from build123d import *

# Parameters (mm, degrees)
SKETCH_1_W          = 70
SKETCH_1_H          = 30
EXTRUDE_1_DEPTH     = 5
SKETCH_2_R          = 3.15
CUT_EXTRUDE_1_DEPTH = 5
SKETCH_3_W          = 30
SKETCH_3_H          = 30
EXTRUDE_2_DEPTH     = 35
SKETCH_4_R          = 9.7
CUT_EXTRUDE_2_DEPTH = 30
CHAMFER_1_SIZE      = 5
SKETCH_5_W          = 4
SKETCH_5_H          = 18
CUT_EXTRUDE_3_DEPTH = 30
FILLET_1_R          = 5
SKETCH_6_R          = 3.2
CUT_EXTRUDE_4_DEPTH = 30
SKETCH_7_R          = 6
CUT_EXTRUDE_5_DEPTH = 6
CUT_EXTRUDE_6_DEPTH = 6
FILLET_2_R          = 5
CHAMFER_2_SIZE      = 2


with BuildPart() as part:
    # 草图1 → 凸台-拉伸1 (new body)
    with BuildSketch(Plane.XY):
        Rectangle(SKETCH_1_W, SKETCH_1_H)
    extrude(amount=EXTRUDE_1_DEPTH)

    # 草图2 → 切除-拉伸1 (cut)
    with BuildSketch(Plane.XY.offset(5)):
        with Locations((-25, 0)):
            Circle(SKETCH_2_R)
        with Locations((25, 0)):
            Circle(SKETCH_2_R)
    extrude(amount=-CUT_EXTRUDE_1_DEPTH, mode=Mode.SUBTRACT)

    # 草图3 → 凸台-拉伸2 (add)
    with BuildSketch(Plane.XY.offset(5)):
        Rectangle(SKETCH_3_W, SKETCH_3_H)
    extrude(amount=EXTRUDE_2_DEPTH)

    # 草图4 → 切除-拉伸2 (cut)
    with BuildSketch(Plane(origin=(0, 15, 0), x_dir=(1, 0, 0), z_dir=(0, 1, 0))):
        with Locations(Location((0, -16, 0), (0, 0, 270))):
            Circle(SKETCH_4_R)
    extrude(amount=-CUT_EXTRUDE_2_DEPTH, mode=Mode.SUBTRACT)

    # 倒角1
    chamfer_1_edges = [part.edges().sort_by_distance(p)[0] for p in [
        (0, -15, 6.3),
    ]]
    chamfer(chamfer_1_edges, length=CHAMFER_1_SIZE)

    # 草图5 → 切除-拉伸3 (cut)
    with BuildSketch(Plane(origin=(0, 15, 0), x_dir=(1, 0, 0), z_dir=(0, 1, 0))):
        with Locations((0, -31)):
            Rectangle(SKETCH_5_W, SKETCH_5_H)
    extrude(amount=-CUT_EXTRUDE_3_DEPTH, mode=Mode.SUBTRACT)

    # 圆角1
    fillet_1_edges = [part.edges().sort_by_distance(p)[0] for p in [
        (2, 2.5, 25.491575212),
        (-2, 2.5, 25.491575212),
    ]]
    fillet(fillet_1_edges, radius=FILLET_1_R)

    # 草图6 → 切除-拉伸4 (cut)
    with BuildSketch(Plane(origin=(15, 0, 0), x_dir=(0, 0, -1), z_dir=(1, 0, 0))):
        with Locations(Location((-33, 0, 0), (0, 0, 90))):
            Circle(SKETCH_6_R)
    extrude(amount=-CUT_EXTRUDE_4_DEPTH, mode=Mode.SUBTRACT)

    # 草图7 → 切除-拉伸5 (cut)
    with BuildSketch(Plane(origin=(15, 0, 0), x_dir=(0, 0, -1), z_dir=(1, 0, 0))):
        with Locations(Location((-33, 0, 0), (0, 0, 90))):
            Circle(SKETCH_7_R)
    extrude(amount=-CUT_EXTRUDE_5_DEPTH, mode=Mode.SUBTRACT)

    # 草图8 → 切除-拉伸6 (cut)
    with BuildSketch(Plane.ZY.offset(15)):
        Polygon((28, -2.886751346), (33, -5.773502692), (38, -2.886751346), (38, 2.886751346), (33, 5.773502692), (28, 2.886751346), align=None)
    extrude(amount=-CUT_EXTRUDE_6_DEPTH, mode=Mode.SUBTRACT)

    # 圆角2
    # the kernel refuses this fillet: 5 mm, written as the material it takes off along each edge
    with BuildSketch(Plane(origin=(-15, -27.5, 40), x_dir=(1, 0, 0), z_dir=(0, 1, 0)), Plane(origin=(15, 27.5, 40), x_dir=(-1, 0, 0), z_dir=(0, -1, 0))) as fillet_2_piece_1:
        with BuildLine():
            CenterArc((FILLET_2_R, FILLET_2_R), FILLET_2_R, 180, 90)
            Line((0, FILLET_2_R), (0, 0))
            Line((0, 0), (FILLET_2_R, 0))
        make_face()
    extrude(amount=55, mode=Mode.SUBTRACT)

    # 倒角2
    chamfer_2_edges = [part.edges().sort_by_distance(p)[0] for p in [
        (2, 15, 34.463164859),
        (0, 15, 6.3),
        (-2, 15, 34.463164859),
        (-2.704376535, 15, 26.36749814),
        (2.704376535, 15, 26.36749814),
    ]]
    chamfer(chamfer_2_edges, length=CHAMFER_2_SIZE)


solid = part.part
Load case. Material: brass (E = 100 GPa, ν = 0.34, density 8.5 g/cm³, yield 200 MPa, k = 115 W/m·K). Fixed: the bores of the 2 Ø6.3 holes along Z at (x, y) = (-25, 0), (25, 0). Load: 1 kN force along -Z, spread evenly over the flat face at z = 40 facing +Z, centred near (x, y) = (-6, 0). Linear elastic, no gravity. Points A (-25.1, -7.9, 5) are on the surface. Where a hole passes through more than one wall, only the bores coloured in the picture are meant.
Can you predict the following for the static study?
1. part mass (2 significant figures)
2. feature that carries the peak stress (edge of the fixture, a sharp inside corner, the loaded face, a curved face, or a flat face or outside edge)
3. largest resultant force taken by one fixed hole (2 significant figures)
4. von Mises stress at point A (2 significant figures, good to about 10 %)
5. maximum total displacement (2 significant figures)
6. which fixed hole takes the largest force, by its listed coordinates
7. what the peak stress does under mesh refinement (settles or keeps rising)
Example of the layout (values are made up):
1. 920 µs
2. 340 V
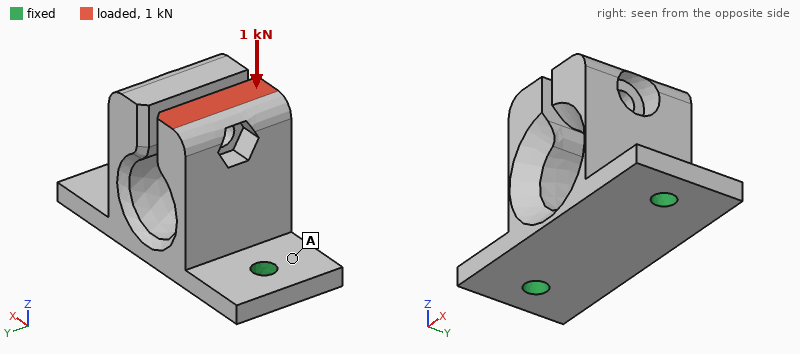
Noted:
1. 240 g
2. edge of the fixture
3. 730 N
4. 11 MPa
5. 78 µm
6. (-25, 0)
7. keeps rising
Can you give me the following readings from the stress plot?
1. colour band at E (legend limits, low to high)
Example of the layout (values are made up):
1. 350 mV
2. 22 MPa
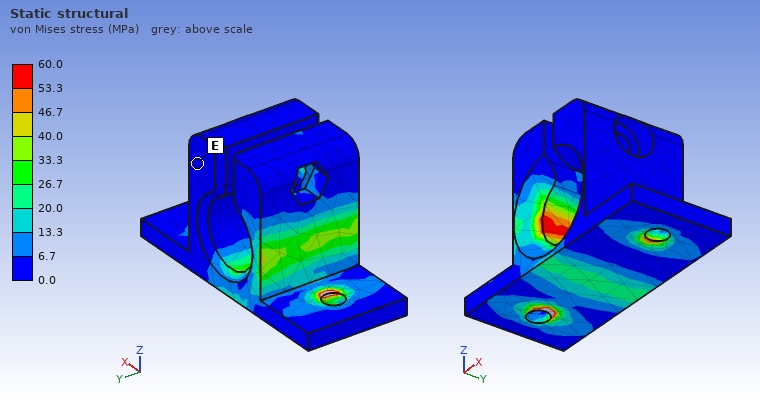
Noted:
1. 0.0 to 6.7 MPa
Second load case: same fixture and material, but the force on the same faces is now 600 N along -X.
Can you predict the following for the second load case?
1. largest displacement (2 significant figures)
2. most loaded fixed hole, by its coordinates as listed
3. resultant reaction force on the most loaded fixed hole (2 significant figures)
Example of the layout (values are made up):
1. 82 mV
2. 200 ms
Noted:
1. 0.18 mm
2. (25, 0)
3. 850 N
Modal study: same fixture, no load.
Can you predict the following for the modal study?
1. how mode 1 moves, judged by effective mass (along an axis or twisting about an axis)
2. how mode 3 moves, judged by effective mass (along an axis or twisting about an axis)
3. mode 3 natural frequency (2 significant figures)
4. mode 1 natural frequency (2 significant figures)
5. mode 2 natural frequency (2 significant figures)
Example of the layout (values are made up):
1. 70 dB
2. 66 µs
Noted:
1. along Y
2. along X
3. 2100 Hz
4. 1600 Hz
5. 1700 Hz
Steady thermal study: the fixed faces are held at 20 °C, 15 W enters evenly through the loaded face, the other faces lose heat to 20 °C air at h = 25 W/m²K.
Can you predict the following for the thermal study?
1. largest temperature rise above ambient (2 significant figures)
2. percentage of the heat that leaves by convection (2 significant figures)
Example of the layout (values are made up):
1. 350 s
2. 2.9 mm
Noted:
1. 29 K
2. 14 %
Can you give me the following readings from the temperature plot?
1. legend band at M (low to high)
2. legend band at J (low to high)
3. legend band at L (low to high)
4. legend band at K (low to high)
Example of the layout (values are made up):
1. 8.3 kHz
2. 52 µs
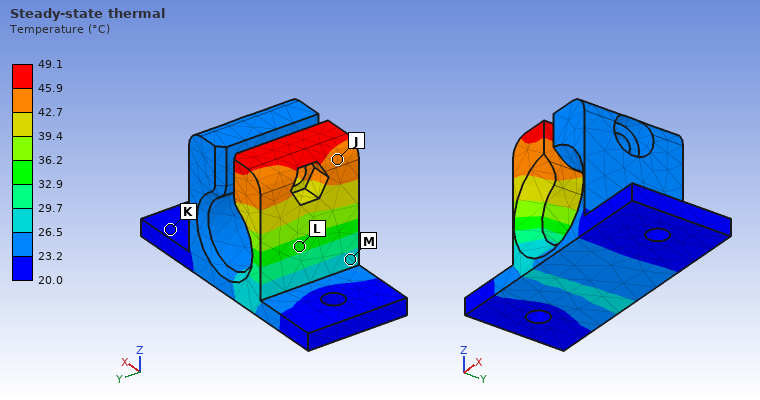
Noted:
1. 26.5 to 29.7 °C
2. 42.7 to 45.9 °C
3. 32.9 to 36.2 °C
4. 20.0 to 23.2 °C
